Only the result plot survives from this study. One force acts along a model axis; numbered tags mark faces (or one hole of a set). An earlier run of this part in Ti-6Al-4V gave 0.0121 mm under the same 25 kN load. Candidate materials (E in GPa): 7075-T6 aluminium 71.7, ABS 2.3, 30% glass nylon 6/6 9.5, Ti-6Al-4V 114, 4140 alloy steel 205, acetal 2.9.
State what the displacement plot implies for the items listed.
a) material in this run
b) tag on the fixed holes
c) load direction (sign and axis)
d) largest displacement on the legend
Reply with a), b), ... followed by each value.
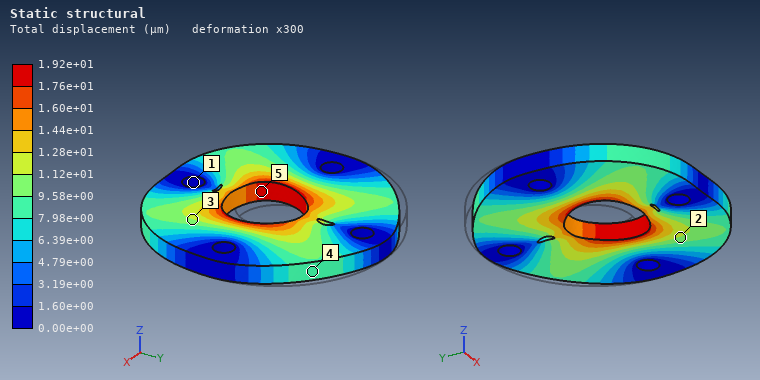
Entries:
a) 7075-T6 aluminium
b) 1
c) -Y
d) 1.92e+01 µm
